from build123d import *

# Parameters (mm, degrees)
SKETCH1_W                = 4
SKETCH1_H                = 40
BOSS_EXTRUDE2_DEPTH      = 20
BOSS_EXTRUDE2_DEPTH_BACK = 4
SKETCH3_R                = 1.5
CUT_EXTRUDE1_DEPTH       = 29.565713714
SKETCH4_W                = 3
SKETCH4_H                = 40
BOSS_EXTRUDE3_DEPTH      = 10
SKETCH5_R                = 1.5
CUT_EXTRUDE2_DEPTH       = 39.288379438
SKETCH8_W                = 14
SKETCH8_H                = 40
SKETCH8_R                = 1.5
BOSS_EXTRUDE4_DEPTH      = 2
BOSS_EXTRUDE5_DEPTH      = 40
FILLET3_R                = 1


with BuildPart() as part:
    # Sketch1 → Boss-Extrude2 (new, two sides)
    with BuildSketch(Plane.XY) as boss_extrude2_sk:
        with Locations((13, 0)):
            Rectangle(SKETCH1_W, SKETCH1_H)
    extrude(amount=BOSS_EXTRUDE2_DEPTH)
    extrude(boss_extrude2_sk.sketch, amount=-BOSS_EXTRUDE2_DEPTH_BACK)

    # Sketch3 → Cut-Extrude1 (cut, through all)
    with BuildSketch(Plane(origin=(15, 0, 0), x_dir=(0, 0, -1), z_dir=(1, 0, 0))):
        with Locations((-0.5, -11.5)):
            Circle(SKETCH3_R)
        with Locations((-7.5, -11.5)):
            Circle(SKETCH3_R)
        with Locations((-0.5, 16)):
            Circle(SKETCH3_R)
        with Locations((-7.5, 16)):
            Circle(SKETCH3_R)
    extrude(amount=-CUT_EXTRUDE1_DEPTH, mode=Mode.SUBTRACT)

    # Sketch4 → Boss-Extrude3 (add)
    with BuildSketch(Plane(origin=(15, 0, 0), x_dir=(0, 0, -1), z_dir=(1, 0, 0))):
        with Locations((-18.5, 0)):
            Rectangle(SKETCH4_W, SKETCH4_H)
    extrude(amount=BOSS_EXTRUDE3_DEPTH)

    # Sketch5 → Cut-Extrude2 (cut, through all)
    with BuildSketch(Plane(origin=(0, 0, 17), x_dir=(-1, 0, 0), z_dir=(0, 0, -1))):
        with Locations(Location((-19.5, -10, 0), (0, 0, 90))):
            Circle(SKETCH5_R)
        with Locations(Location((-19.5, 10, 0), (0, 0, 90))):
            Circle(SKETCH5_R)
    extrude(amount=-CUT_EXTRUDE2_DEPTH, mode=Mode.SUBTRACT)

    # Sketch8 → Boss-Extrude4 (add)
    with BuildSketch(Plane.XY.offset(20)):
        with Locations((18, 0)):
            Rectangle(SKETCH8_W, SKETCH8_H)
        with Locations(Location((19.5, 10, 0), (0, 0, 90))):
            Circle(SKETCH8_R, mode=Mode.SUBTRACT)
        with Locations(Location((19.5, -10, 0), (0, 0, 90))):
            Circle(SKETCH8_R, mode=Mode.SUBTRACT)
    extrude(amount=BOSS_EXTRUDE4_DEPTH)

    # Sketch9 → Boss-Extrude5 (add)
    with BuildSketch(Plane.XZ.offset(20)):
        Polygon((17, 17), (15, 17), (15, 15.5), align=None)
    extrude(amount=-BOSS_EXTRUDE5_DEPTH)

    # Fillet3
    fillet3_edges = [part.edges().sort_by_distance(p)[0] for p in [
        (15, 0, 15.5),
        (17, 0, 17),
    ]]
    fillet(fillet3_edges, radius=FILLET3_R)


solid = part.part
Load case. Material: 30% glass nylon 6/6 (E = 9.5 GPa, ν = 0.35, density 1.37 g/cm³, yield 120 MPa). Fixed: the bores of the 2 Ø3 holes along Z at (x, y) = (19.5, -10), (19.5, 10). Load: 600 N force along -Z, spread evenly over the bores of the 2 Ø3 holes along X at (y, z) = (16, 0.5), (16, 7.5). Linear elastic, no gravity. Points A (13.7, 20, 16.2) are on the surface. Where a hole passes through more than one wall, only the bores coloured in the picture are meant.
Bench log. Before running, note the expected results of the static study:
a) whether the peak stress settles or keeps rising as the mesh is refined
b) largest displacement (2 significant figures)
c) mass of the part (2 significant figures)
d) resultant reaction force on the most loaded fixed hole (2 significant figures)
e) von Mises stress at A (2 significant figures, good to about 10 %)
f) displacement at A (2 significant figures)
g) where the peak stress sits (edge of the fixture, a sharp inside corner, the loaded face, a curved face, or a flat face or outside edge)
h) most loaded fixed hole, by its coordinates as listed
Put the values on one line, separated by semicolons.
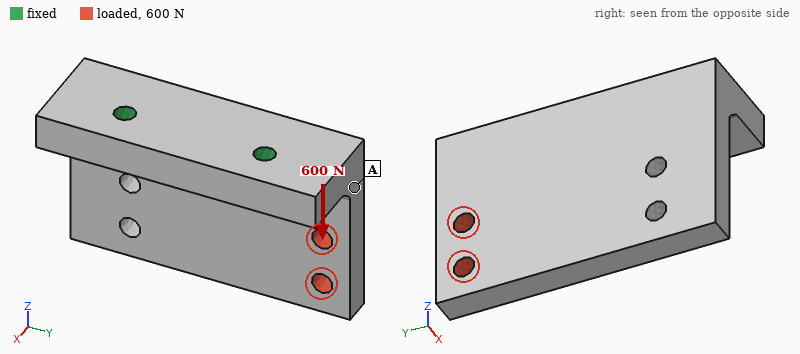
keeps rising; 0.25 mm; 8.3 g; 700 N; 12 MPa; 0.099 mm; edge of the fixture; (19.5, 10)
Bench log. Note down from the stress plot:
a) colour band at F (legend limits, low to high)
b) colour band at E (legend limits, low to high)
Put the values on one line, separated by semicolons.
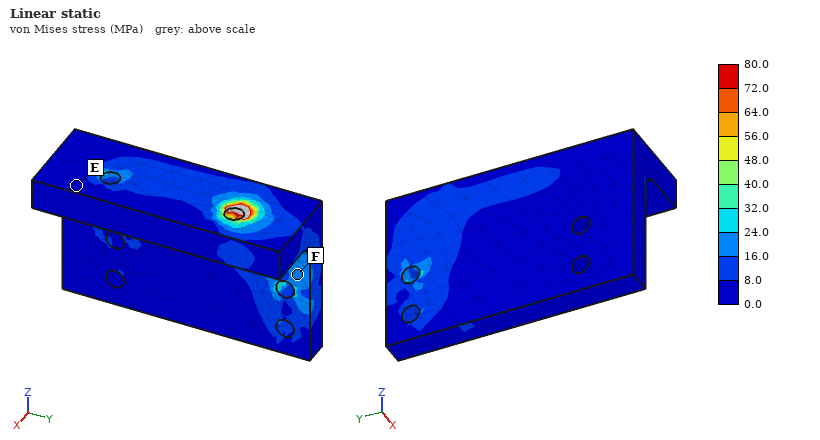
16.0 to 24.0 MPa; 0.0 to 8.0 MPa
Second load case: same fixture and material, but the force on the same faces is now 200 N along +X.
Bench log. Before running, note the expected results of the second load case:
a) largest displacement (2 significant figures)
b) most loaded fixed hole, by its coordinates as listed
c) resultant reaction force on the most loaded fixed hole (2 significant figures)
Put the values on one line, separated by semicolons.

0.50 mm; (19.5, 10); 250 N
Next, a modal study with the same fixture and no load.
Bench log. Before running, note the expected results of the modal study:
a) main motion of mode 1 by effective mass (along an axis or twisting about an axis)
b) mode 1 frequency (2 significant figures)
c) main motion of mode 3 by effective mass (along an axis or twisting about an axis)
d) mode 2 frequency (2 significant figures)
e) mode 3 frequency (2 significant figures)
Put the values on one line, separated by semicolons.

along X; 2800 Hz; along Y; 4600 Hz; 7200 Hz
